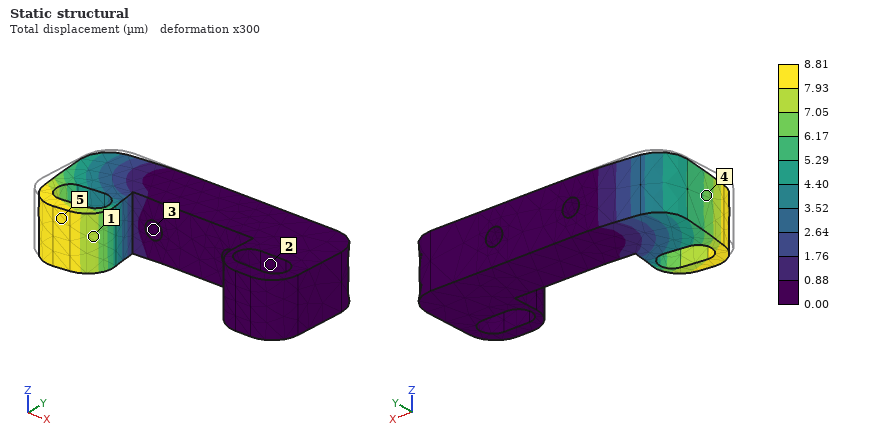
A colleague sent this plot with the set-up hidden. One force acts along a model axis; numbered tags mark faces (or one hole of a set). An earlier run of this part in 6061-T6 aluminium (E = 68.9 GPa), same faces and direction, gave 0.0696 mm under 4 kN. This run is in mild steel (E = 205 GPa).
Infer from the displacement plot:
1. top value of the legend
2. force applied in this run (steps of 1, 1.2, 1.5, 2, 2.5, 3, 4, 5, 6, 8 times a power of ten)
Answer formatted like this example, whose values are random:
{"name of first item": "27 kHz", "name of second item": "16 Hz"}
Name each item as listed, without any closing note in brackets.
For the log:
{"top value of the legend": "8.81 µm", "force applied in this run": "1.5 kN"}
